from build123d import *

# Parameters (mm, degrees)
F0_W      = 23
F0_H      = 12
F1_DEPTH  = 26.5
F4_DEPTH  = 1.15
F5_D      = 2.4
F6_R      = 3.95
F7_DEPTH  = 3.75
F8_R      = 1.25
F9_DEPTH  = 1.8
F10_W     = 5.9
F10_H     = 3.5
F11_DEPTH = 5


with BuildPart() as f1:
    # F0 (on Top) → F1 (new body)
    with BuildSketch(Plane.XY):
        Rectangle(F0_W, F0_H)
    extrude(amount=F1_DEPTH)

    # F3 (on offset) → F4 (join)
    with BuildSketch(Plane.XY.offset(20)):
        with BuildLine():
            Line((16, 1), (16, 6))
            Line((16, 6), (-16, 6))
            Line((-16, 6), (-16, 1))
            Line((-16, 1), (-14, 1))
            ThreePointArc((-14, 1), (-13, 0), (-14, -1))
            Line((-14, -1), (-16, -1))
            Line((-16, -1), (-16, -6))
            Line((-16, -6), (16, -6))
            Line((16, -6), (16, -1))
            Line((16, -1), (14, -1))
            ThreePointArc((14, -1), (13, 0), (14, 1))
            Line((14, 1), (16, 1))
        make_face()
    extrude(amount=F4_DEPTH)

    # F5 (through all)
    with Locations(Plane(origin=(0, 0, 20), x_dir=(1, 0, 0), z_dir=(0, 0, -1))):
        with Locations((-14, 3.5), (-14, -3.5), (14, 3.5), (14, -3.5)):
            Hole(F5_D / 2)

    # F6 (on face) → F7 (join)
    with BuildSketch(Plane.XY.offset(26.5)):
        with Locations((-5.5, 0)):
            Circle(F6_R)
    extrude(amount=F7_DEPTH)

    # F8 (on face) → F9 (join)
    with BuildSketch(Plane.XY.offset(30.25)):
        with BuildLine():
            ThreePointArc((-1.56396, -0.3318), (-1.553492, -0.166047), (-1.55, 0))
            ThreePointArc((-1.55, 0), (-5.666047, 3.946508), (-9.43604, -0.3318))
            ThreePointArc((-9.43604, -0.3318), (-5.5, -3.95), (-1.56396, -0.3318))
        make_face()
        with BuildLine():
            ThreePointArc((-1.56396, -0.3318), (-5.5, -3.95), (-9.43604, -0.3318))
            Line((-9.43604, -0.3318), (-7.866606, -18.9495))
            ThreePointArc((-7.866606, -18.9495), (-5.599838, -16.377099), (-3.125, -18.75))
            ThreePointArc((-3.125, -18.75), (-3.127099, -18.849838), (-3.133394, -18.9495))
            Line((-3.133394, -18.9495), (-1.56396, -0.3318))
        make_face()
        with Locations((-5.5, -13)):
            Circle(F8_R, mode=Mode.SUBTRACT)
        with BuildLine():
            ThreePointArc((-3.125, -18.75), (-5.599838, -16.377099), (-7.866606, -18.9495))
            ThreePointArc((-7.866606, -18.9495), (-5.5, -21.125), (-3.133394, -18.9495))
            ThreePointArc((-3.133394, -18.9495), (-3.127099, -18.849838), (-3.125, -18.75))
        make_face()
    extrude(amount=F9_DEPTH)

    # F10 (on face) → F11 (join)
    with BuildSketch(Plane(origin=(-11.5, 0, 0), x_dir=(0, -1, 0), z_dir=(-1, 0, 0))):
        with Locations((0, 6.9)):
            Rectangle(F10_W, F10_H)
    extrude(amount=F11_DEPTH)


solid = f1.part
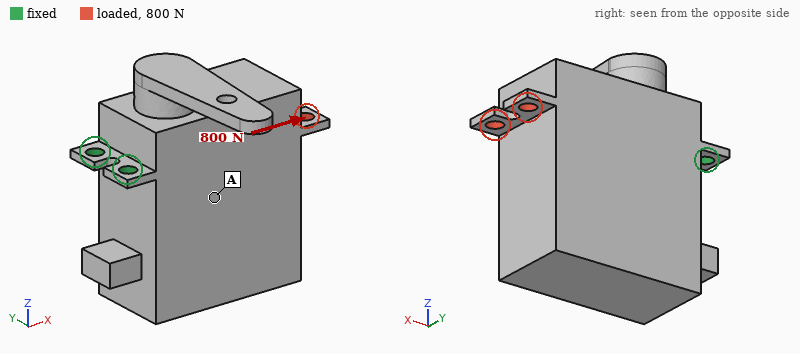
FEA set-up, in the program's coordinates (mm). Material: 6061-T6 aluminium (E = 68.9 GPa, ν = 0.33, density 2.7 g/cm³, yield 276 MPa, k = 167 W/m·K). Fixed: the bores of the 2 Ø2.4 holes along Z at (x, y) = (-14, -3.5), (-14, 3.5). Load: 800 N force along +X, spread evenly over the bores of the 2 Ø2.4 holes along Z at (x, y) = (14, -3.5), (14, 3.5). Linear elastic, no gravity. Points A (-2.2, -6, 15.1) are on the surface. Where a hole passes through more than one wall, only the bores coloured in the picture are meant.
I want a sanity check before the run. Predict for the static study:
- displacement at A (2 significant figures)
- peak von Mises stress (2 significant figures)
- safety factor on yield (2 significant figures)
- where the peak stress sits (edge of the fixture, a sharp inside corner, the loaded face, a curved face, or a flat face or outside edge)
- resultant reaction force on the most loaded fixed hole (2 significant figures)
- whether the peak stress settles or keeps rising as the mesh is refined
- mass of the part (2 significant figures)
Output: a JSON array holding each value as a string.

["3.7 µm", "220 MPa", "1.2", "the loaded face", "400 N", "settles", "21 g"]
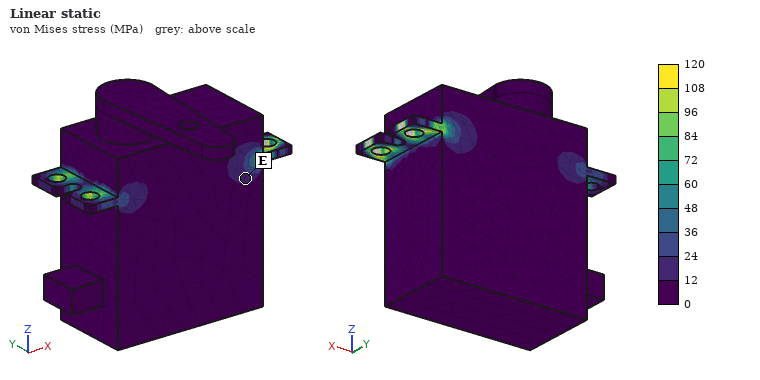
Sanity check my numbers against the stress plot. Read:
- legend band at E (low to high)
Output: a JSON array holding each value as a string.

["12 to 24 MPa"]
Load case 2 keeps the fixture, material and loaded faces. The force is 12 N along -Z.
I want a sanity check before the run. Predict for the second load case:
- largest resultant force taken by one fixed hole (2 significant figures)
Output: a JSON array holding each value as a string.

["6.0 N"]
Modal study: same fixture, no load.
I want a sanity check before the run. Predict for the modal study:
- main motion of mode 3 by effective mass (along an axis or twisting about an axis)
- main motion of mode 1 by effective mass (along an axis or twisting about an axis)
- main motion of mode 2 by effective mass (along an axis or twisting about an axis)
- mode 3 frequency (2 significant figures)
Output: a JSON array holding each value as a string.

["along Y", "along Z", "along Y", "4800 Hz"]
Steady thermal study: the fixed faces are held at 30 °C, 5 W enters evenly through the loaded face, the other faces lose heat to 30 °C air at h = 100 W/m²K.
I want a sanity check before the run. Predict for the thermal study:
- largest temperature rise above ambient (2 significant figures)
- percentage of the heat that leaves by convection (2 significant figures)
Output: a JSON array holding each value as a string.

["19 K", "33 %"]
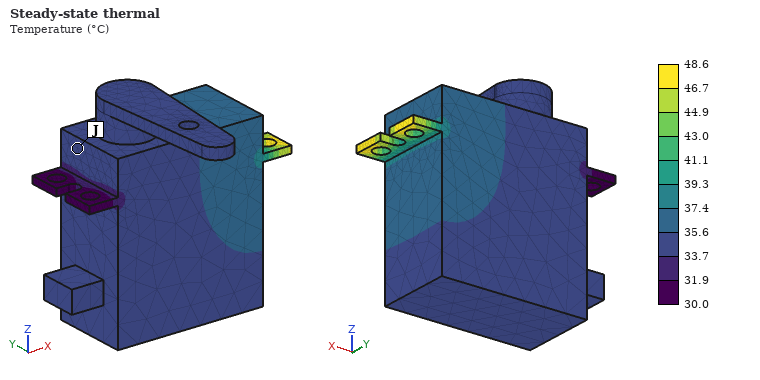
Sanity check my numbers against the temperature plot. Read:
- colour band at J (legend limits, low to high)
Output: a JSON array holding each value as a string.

["33.7 to 35.6 °C"]
